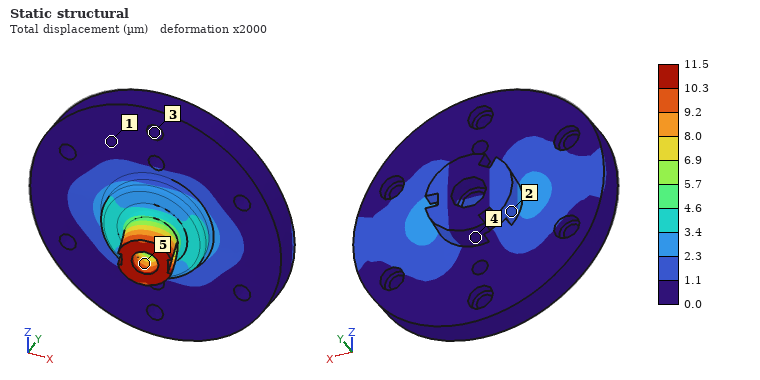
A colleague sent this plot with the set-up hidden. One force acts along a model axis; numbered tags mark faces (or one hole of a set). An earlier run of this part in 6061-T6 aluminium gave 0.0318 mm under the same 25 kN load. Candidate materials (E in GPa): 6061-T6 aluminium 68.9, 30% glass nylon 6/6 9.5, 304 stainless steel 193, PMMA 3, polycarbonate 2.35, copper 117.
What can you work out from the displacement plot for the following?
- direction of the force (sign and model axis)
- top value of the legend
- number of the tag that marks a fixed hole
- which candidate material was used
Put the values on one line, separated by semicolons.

+X; 11.5 µm; 3; 304 stainless steel
